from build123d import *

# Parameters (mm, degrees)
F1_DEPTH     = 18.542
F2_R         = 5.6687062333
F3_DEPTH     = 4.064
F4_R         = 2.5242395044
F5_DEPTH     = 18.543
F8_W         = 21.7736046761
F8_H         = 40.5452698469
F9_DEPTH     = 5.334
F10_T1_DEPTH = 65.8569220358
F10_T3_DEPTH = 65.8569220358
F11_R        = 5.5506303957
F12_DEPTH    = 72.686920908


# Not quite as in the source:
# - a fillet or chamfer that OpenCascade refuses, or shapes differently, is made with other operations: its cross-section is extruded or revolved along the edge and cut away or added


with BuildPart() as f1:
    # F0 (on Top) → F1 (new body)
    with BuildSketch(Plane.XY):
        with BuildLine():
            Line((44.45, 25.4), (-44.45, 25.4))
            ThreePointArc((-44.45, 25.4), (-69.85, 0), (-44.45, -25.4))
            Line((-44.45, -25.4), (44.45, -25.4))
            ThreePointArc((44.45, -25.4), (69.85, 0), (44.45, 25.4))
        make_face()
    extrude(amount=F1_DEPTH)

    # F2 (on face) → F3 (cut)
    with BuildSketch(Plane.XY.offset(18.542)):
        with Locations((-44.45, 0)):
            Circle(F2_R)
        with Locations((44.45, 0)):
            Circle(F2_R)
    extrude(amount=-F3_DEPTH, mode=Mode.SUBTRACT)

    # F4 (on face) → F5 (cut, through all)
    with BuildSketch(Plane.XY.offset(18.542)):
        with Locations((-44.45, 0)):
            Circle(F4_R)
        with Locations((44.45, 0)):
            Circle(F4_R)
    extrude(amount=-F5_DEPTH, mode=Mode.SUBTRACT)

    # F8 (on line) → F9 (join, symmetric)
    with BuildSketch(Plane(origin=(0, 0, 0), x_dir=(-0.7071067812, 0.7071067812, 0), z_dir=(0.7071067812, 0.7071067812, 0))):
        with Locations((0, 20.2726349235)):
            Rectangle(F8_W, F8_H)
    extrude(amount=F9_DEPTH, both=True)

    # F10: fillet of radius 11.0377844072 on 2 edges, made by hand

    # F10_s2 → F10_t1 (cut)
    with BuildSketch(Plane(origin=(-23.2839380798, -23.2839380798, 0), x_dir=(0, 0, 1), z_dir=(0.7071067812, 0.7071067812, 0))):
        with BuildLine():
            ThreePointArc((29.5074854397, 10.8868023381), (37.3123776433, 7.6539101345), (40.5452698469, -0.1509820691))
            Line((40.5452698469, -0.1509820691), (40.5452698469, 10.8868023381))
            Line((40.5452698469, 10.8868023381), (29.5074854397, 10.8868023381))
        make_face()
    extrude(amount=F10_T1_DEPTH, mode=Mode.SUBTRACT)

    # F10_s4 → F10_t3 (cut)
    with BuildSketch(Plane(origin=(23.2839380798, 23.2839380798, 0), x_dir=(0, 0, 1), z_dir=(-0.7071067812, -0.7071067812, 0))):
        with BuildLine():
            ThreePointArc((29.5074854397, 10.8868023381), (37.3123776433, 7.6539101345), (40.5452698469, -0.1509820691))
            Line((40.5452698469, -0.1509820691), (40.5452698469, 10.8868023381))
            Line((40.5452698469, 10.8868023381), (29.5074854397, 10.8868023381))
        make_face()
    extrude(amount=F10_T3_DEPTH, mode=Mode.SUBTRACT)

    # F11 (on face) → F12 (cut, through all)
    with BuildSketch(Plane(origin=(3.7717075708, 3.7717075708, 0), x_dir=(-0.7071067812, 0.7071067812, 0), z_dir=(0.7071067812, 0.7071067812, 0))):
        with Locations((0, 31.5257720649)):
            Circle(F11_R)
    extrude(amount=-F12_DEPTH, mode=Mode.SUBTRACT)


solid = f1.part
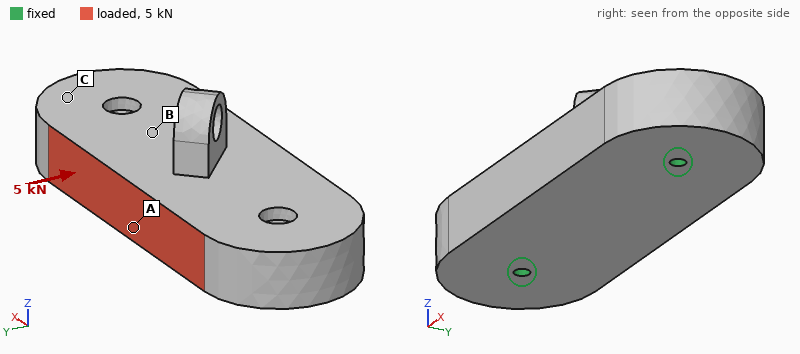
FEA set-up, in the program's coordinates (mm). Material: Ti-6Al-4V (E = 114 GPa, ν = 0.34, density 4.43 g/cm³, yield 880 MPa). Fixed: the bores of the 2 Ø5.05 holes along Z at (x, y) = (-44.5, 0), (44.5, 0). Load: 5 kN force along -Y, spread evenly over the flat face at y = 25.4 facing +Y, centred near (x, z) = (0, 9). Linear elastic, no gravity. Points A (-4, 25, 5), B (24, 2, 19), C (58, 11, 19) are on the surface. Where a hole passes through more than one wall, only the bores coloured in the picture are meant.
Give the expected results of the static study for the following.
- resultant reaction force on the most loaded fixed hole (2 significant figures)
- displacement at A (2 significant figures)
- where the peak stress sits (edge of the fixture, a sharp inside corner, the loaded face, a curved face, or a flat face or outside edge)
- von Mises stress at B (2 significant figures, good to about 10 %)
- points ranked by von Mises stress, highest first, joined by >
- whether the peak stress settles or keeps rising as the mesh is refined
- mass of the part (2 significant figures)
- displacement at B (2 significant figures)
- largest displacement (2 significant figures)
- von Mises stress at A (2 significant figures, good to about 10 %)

2.5 kN
3.9 µm
edge of the fixture
3.9 MPa
A > B > C
keeps rising
550 g
3.1 µm
5.3 µm
6.5 MPa
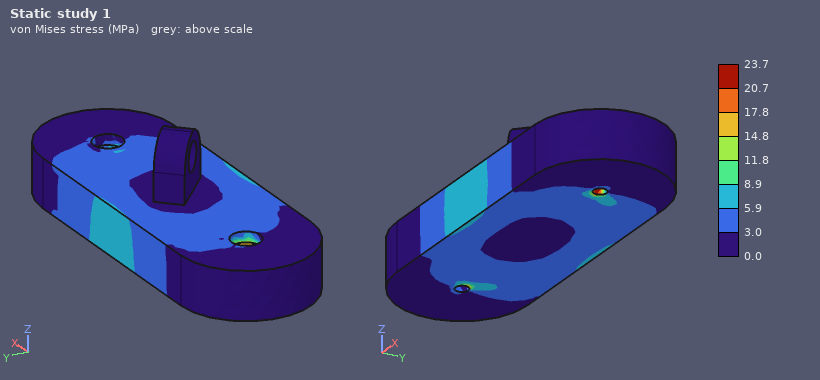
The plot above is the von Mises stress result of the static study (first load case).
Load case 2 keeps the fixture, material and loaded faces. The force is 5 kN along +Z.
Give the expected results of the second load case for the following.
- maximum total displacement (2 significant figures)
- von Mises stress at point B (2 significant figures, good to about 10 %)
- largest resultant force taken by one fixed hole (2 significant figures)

35 µm
16 MPa
2.6 kN
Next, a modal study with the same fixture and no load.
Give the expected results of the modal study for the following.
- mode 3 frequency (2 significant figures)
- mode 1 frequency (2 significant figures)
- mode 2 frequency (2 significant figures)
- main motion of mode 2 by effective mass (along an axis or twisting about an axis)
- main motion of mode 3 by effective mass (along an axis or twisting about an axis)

9800 Hz
6100 Hz
6400 Hz
along Z
along Y
